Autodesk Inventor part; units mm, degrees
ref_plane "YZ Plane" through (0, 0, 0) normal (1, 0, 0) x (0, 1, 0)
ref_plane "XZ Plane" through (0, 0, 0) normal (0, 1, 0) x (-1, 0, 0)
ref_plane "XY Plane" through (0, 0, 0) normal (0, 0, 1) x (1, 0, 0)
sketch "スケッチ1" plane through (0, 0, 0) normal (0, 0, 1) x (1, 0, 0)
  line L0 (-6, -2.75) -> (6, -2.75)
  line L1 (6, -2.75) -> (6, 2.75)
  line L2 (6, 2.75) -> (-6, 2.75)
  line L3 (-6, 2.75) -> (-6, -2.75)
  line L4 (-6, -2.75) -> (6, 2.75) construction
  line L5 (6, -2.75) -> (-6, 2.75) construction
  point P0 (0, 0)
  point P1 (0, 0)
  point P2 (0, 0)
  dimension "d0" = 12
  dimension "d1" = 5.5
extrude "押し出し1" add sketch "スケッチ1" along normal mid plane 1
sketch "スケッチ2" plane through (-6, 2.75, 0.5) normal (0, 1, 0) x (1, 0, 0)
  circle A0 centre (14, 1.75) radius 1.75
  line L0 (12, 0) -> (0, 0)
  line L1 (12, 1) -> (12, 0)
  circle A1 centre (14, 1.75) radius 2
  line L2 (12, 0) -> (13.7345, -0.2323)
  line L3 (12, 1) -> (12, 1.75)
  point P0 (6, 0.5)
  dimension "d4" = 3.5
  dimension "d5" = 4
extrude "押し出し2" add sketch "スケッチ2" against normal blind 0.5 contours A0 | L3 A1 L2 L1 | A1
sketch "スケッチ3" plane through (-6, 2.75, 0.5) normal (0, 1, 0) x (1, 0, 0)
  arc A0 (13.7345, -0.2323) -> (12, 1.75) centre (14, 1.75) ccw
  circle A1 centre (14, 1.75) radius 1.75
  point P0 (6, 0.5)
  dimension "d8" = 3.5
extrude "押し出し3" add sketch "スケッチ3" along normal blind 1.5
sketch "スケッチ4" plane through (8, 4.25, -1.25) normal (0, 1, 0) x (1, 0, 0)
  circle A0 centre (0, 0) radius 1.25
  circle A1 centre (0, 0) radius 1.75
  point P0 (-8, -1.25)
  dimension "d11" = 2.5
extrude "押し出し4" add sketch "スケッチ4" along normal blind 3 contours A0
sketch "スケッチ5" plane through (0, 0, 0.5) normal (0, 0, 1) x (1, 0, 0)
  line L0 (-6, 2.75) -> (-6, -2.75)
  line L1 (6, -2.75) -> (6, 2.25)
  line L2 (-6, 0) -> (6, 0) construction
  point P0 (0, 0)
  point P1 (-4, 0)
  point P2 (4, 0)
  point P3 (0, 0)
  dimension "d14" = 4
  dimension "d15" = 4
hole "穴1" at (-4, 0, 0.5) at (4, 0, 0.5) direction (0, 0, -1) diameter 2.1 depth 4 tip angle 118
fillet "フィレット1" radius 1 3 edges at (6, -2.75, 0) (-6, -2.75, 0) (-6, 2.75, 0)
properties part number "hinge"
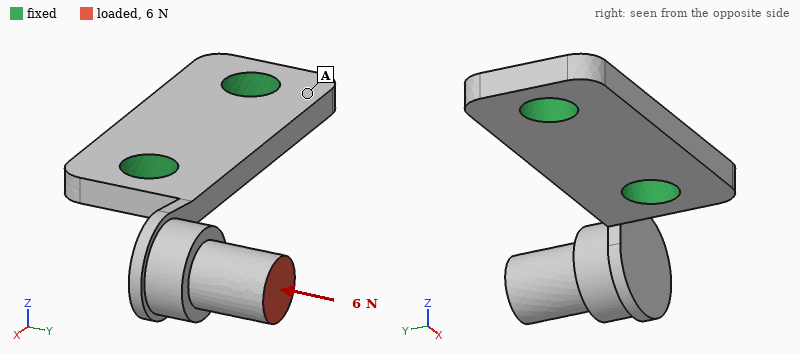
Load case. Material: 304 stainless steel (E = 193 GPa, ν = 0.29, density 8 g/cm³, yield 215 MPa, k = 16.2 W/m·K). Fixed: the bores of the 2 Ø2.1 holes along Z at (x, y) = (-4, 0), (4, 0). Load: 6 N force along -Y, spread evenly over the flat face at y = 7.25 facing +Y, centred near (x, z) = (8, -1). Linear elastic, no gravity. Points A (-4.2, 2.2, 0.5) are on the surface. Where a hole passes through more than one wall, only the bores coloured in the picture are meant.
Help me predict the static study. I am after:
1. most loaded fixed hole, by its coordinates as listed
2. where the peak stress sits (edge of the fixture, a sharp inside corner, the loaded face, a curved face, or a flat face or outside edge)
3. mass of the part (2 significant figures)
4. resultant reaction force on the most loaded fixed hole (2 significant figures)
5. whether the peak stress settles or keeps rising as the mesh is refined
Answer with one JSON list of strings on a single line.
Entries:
["(4, 0)", "a sharp inside corner", "0.75 g", "7.3 N", "keeps rising"]
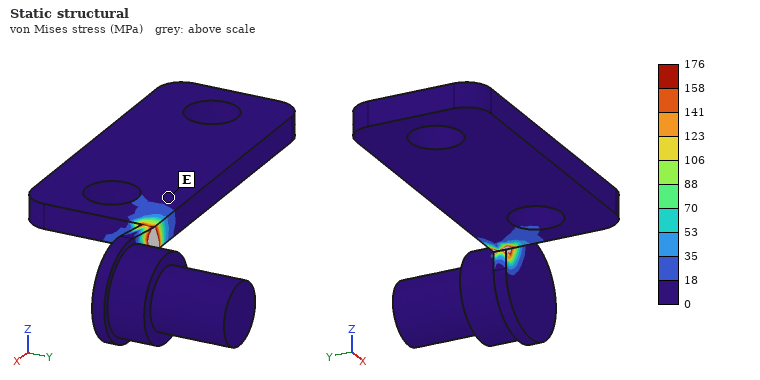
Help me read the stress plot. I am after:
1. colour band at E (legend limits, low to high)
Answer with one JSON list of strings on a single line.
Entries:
["0 to 18 MPa"]
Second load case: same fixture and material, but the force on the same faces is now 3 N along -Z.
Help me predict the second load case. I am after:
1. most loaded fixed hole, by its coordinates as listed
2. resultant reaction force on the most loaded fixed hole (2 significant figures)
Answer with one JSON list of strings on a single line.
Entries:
["(4, 0)", "3.3 N"]
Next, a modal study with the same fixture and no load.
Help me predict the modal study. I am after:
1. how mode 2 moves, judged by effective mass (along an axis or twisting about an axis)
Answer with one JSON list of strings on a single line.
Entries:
["along Z"]
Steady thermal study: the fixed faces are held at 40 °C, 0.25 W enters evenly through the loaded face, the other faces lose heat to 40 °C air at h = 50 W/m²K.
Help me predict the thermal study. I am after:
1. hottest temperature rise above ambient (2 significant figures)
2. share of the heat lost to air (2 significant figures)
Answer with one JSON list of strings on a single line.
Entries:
["39 K", "43 %"]
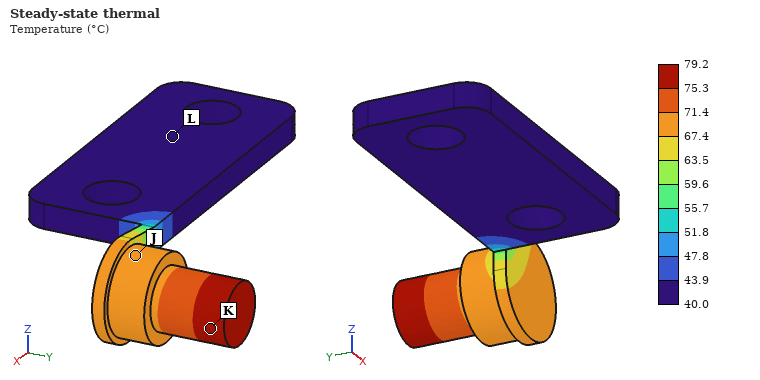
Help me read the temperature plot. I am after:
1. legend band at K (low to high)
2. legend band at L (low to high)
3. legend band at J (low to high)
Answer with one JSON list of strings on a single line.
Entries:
["75.3 to 79.2 °C", "40.0 to 43.9 °C", "67.4 to 71.4 °C"]
